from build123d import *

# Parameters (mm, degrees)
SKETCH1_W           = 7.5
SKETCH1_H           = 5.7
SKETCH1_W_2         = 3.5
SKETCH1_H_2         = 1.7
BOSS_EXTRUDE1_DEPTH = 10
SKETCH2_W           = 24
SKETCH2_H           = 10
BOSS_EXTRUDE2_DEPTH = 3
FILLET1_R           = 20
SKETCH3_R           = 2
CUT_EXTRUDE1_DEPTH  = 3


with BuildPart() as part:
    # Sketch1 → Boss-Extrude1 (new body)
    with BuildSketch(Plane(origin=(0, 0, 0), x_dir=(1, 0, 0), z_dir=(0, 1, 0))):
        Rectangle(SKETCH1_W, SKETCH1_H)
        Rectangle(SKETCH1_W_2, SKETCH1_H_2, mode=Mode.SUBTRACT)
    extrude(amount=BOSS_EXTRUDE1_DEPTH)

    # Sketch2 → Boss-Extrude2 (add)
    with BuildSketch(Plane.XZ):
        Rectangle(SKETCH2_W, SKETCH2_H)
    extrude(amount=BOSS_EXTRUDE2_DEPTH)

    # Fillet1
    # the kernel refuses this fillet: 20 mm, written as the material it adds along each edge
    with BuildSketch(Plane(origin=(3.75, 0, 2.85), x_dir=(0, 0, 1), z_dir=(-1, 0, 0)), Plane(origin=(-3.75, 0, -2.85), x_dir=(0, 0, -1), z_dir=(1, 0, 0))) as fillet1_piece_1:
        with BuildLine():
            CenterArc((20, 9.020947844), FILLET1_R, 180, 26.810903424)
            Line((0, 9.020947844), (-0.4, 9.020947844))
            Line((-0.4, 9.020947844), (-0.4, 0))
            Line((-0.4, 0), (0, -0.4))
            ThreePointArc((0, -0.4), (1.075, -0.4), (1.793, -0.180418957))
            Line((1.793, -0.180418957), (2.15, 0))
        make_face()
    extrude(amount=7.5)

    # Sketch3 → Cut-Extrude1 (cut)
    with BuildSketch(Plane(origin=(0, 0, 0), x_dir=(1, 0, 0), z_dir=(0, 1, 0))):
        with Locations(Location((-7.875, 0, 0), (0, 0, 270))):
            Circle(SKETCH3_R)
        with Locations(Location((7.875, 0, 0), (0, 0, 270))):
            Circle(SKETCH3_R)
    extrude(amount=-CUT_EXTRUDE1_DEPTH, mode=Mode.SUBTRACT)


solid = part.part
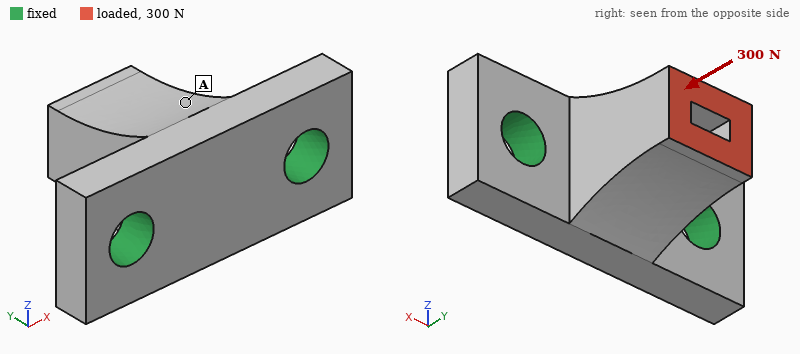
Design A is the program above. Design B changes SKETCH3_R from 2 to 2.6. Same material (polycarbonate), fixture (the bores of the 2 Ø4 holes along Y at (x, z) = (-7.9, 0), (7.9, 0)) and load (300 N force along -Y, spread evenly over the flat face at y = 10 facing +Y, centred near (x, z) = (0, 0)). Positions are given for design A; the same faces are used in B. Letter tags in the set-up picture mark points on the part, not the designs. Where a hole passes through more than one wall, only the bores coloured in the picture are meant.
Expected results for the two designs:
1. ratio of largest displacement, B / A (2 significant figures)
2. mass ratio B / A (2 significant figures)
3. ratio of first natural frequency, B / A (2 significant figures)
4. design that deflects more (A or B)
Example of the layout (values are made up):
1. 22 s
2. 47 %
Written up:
1. 0.82
2. 0.95
3. 1.1
4. A
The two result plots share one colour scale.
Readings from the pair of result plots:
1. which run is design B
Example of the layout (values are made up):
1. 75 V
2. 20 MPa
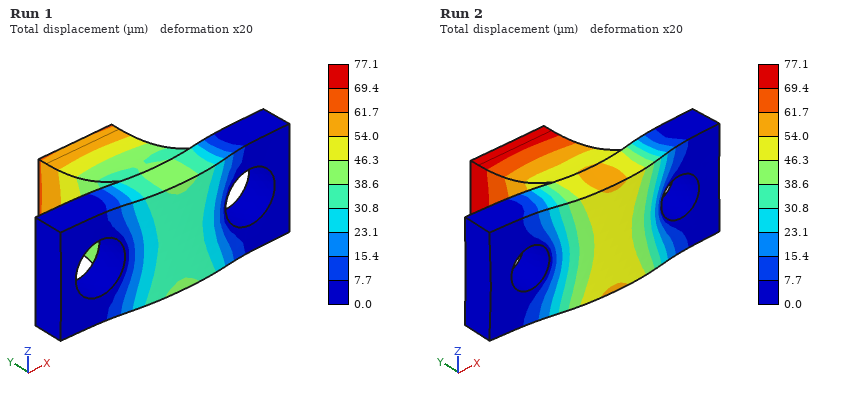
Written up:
1. Run 1
